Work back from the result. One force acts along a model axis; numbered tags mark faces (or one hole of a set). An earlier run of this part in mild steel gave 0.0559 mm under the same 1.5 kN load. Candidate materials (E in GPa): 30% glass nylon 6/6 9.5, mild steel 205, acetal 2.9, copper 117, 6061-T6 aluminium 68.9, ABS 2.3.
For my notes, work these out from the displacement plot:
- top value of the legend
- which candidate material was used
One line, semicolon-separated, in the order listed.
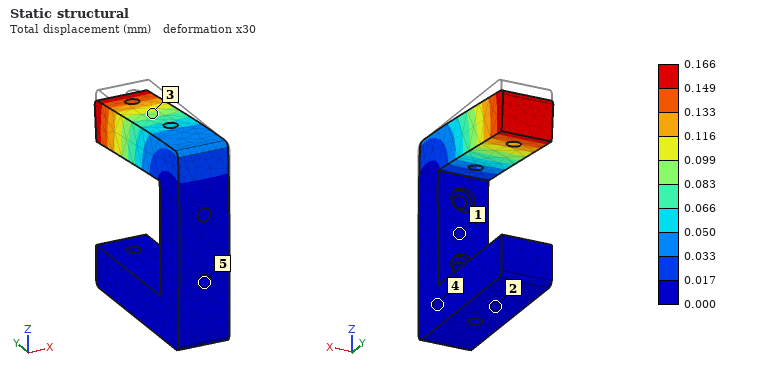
0.166 mm; 6061-T6 aluminium
